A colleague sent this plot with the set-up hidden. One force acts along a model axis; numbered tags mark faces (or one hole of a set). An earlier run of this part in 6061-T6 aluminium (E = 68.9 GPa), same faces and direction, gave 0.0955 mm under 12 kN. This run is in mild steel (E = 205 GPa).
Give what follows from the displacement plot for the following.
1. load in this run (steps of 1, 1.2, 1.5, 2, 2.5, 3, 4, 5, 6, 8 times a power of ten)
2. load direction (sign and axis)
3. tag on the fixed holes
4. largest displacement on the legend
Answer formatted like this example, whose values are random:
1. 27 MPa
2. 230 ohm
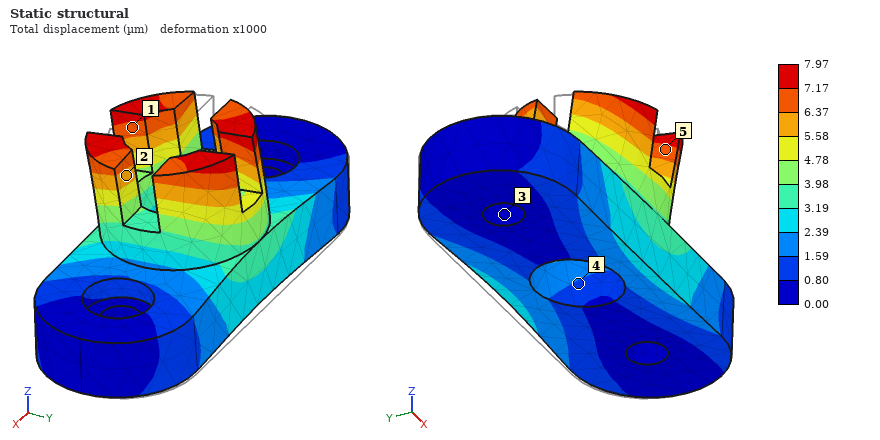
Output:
1. 3 kN
2. -Y
3. 3
4. 7.97 µm
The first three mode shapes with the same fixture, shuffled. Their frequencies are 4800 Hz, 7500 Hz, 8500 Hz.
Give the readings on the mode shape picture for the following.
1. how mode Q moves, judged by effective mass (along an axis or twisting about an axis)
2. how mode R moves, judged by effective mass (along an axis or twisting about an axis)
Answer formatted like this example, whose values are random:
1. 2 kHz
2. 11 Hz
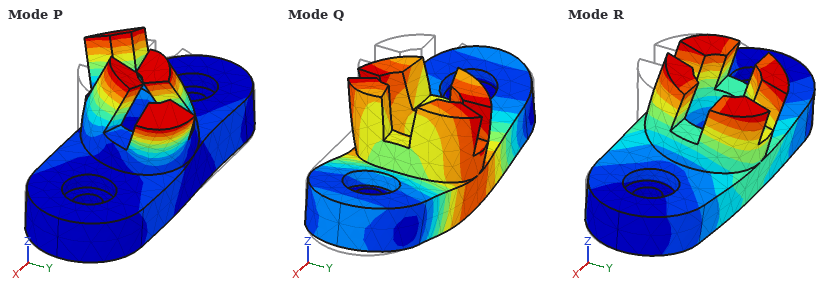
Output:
1. along Z
2. along Y
